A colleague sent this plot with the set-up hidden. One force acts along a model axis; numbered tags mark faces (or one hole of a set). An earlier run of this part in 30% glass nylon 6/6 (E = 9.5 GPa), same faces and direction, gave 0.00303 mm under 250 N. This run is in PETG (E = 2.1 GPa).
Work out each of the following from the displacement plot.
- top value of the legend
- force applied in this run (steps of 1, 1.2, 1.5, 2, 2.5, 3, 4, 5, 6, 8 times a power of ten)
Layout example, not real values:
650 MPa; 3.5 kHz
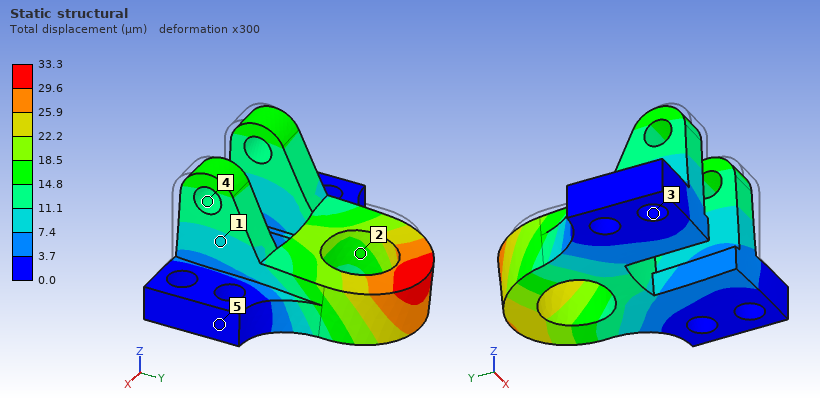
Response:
33.3 µm; 600 N
